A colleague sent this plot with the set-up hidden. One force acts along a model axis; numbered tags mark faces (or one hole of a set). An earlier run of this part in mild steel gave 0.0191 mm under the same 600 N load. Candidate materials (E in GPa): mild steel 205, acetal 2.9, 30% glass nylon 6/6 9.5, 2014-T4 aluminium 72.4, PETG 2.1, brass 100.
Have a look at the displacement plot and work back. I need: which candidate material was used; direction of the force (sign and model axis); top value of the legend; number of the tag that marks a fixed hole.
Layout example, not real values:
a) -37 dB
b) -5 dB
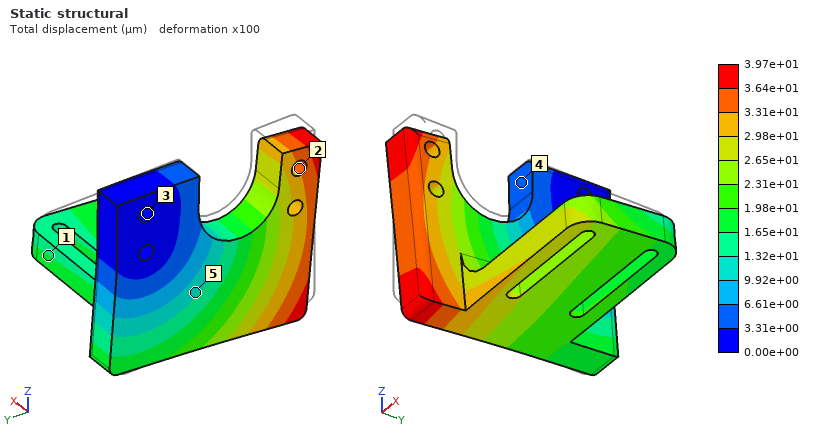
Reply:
a) brass
b) -Z
c) 3.97e+01 µm
d) 3
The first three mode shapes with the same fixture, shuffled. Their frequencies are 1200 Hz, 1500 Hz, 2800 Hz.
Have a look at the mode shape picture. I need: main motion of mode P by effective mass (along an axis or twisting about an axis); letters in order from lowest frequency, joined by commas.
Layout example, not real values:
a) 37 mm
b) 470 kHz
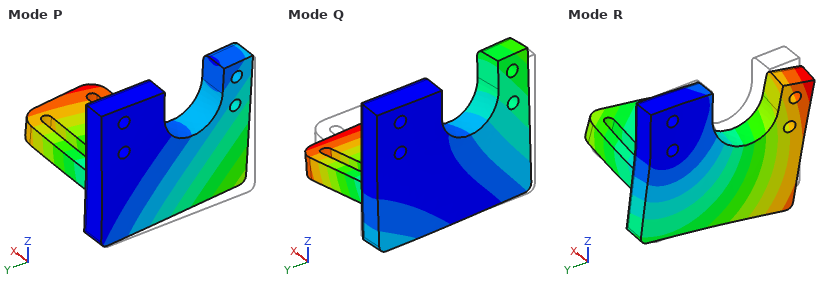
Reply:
a) along X
b) P, Q, R
